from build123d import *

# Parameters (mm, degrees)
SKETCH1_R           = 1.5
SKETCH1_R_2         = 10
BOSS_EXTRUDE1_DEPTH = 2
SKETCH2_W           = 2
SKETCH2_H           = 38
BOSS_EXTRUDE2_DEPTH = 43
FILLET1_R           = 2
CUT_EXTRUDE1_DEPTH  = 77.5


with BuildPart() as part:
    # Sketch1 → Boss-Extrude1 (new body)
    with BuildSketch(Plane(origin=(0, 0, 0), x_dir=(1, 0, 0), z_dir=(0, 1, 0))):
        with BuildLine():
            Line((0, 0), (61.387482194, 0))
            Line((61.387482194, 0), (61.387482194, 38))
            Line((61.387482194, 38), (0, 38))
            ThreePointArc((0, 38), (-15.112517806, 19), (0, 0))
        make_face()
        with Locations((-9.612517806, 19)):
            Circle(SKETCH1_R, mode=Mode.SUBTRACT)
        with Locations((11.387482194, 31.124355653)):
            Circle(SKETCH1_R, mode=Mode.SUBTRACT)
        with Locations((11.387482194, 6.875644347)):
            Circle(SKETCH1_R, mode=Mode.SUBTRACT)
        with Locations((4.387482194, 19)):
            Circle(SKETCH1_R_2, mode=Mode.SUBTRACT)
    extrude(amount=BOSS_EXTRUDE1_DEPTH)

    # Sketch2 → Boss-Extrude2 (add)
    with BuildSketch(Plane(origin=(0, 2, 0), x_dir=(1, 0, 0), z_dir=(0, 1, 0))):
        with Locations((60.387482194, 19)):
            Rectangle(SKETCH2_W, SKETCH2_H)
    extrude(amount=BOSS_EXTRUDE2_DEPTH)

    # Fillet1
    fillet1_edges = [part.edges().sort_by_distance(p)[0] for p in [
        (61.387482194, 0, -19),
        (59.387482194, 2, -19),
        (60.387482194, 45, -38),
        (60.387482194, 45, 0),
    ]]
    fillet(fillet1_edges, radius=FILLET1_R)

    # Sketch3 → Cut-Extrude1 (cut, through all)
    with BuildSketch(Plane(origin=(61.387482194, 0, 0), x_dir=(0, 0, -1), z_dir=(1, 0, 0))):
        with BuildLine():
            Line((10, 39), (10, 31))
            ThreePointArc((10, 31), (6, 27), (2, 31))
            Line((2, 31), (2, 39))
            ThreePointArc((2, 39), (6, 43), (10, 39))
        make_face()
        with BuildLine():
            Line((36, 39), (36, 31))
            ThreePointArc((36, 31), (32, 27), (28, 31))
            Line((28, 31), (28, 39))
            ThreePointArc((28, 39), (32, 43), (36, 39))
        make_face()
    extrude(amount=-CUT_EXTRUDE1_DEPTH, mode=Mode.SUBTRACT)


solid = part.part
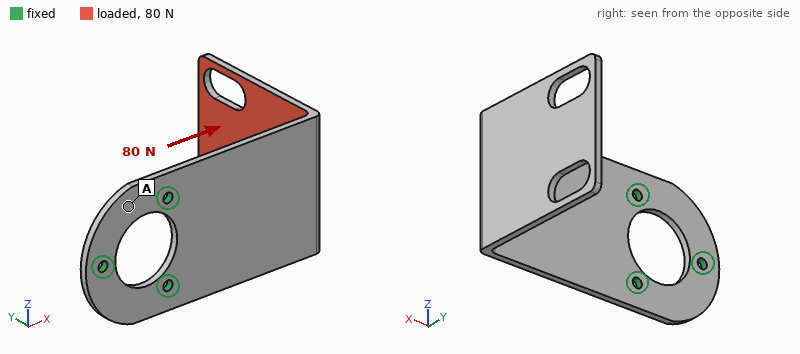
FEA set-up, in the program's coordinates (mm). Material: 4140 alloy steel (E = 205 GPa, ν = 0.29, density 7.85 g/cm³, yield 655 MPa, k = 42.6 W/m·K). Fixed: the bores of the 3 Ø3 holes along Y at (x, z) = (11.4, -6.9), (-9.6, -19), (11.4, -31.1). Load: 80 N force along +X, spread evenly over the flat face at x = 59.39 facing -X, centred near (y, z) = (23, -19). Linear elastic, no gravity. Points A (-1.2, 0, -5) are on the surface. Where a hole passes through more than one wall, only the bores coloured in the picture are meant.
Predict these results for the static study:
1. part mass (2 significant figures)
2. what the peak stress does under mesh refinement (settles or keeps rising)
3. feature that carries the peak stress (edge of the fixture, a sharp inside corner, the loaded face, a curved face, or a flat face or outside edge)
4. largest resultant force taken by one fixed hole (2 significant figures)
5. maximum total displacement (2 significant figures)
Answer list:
60 g
keeps rising
edge of the fixture
40 N
0.95 mm
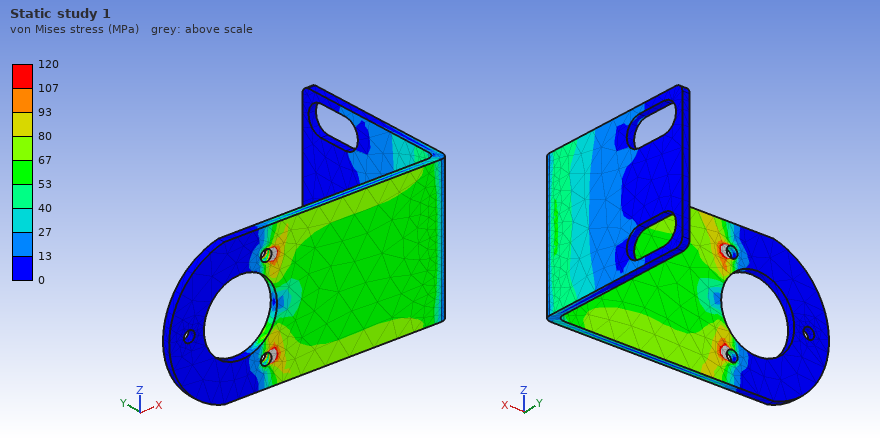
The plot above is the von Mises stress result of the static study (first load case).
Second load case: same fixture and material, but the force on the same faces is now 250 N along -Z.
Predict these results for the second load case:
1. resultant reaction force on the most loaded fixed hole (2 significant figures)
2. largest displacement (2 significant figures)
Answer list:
480 N
1.2 mm
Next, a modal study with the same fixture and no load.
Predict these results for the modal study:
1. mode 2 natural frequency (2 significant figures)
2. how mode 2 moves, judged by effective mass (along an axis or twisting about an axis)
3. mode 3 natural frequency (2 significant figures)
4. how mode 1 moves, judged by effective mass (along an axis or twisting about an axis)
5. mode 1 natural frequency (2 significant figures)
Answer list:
590 Hz
along Z
830 Hz
along Y
270 Hz
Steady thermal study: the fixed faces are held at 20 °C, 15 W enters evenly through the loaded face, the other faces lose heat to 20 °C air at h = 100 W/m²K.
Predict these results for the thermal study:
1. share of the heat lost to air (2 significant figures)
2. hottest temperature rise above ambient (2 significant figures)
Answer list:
95 %
62 K
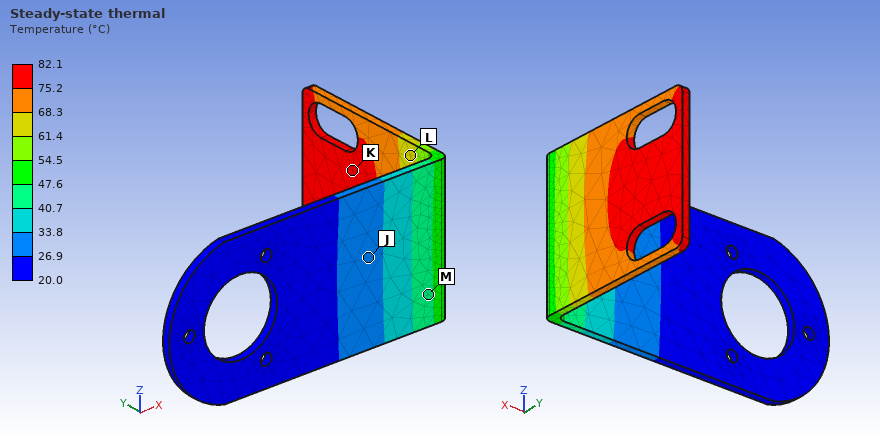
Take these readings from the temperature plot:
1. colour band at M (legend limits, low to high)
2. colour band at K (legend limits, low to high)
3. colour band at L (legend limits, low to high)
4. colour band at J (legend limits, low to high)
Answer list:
40.7 to 47.6 °C
75.2 to 82.1 °C
61.4 to 68.3 °C
26.9 to 33.8 °C
